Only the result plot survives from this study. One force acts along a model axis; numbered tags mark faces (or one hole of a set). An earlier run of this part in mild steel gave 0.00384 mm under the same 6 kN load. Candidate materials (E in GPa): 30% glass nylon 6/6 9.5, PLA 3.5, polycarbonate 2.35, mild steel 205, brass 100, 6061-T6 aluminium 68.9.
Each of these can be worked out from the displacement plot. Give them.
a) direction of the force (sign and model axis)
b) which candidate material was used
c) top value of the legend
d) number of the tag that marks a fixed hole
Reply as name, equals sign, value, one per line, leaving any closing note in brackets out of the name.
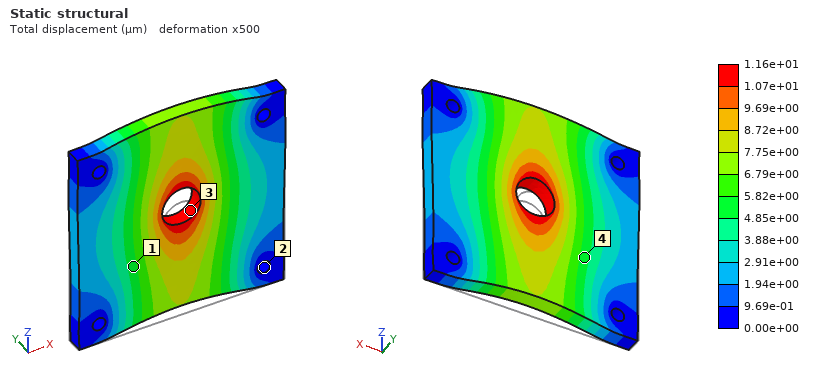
direction of the force = +Z
which candidate material was used = 6061-T6 aluminium
top value of the legend = 1.16e+01 µm
number of the tag that marks a fixed hole = 2
